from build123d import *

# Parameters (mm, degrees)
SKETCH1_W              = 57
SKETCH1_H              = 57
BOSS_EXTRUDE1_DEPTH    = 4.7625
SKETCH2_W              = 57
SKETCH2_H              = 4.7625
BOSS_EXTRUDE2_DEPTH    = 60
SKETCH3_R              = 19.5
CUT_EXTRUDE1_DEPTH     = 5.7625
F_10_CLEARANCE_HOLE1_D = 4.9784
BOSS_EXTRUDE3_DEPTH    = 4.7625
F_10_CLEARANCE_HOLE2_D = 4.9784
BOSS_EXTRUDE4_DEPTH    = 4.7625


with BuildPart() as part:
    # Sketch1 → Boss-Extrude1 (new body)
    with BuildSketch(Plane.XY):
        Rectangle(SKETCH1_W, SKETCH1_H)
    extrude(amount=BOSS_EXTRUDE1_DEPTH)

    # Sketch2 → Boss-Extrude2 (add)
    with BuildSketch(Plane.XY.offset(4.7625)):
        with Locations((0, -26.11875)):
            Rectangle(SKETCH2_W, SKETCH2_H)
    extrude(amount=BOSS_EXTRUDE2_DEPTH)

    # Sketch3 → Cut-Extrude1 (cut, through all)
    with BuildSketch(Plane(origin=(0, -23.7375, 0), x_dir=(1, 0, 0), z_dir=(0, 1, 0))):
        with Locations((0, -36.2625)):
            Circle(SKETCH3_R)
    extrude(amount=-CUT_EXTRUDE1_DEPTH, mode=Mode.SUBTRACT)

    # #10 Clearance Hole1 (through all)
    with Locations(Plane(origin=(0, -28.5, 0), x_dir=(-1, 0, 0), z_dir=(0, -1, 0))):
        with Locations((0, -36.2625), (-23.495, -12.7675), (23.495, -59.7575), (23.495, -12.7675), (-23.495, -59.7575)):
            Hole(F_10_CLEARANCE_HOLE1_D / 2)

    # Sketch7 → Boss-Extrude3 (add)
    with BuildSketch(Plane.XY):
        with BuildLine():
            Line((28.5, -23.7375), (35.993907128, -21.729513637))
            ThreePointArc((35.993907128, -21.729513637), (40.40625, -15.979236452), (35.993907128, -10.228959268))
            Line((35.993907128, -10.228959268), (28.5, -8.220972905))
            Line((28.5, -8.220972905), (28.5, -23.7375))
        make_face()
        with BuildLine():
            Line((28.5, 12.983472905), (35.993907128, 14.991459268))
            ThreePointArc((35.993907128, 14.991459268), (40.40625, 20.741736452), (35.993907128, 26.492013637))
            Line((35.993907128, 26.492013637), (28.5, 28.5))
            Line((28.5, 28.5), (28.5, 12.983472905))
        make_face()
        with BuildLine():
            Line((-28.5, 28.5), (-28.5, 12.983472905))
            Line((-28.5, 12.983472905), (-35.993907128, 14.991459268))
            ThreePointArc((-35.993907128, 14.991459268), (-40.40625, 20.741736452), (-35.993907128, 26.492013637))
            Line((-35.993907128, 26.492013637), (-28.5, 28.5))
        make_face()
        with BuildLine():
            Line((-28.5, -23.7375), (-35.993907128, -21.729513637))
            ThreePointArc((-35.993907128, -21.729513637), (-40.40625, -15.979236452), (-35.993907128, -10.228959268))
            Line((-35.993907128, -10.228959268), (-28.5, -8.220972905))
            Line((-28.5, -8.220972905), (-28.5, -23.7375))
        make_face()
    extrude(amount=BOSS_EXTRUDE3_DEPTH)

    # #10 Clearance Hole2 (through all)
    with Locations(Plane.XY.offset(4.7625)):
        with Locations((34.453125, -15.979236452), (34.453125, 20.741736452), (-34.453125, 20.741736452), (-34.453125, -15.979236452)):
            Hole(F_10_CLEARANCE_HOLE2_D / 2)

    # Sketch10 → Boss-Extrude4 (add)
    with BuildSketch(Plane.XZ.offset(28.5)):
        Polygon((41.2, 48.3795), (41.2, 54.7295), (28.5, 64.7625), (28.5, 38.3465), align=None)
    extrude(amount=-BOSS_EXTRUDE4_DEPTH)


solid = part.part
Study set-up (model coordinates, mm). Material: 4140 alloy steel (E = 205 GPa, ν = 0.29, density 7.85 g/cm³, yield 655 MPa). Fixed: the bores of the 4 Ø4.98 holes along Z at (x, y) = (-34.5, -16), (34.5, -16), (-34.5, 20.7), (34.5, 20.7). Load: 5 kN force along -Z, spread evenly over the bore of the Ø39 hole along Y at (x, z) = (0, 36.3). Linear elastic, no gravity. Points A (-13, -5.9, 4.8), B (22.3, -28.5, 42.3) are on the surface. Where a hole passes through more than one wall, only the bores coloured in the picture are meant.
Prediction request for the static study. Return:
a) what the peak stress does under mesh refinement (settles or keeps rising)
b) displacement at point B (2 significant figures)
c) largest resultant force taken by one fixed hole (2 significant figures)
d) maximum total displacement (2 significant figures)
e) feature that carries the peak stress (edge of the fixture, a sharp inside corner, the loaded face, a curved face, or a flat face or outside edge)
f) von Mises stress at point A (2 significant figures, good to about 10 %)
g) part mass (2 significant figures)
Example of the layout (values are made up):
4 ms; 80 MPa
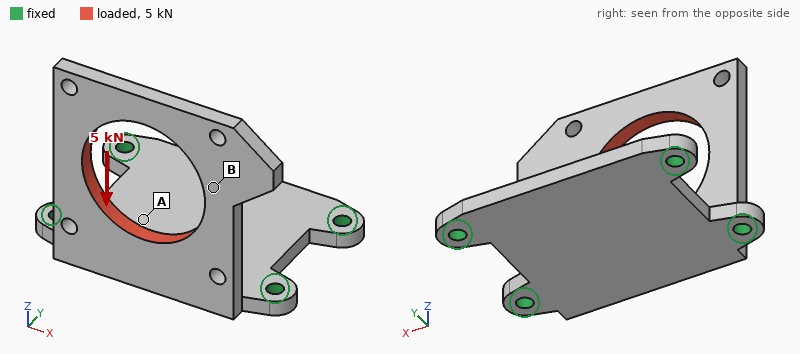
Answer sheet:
keeps rising; 0.19 mm; 2.9 kN; 0.29 mm; edge of the fixture; 64 MPa; 230 g
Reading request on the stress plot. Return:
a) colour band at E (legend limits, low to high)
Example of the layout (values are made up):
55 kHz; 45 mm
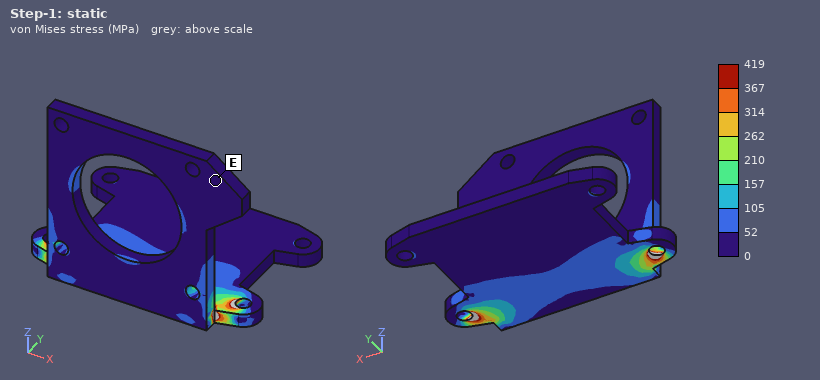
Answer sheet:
0 to 52 MPa
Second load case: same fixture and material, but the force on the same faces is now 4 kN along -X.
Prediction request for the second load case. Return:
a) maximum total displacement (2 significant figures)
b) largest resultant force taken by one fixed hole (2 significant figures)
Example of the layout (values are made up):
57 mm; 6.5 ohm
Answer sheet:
0.19 mm; 3.1 kN
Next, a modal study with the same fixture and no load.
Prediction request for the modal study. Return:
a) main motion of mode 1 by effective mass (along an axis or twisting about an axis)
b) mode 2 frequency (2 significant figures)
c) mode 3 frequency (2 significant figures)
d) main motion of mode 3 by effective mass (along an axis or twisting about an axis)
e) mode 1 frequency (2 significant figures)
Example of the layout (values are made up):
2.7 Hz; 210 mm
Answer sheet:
along Y; 1600 Hz; 2900 Hz; along X; 700 Hz
